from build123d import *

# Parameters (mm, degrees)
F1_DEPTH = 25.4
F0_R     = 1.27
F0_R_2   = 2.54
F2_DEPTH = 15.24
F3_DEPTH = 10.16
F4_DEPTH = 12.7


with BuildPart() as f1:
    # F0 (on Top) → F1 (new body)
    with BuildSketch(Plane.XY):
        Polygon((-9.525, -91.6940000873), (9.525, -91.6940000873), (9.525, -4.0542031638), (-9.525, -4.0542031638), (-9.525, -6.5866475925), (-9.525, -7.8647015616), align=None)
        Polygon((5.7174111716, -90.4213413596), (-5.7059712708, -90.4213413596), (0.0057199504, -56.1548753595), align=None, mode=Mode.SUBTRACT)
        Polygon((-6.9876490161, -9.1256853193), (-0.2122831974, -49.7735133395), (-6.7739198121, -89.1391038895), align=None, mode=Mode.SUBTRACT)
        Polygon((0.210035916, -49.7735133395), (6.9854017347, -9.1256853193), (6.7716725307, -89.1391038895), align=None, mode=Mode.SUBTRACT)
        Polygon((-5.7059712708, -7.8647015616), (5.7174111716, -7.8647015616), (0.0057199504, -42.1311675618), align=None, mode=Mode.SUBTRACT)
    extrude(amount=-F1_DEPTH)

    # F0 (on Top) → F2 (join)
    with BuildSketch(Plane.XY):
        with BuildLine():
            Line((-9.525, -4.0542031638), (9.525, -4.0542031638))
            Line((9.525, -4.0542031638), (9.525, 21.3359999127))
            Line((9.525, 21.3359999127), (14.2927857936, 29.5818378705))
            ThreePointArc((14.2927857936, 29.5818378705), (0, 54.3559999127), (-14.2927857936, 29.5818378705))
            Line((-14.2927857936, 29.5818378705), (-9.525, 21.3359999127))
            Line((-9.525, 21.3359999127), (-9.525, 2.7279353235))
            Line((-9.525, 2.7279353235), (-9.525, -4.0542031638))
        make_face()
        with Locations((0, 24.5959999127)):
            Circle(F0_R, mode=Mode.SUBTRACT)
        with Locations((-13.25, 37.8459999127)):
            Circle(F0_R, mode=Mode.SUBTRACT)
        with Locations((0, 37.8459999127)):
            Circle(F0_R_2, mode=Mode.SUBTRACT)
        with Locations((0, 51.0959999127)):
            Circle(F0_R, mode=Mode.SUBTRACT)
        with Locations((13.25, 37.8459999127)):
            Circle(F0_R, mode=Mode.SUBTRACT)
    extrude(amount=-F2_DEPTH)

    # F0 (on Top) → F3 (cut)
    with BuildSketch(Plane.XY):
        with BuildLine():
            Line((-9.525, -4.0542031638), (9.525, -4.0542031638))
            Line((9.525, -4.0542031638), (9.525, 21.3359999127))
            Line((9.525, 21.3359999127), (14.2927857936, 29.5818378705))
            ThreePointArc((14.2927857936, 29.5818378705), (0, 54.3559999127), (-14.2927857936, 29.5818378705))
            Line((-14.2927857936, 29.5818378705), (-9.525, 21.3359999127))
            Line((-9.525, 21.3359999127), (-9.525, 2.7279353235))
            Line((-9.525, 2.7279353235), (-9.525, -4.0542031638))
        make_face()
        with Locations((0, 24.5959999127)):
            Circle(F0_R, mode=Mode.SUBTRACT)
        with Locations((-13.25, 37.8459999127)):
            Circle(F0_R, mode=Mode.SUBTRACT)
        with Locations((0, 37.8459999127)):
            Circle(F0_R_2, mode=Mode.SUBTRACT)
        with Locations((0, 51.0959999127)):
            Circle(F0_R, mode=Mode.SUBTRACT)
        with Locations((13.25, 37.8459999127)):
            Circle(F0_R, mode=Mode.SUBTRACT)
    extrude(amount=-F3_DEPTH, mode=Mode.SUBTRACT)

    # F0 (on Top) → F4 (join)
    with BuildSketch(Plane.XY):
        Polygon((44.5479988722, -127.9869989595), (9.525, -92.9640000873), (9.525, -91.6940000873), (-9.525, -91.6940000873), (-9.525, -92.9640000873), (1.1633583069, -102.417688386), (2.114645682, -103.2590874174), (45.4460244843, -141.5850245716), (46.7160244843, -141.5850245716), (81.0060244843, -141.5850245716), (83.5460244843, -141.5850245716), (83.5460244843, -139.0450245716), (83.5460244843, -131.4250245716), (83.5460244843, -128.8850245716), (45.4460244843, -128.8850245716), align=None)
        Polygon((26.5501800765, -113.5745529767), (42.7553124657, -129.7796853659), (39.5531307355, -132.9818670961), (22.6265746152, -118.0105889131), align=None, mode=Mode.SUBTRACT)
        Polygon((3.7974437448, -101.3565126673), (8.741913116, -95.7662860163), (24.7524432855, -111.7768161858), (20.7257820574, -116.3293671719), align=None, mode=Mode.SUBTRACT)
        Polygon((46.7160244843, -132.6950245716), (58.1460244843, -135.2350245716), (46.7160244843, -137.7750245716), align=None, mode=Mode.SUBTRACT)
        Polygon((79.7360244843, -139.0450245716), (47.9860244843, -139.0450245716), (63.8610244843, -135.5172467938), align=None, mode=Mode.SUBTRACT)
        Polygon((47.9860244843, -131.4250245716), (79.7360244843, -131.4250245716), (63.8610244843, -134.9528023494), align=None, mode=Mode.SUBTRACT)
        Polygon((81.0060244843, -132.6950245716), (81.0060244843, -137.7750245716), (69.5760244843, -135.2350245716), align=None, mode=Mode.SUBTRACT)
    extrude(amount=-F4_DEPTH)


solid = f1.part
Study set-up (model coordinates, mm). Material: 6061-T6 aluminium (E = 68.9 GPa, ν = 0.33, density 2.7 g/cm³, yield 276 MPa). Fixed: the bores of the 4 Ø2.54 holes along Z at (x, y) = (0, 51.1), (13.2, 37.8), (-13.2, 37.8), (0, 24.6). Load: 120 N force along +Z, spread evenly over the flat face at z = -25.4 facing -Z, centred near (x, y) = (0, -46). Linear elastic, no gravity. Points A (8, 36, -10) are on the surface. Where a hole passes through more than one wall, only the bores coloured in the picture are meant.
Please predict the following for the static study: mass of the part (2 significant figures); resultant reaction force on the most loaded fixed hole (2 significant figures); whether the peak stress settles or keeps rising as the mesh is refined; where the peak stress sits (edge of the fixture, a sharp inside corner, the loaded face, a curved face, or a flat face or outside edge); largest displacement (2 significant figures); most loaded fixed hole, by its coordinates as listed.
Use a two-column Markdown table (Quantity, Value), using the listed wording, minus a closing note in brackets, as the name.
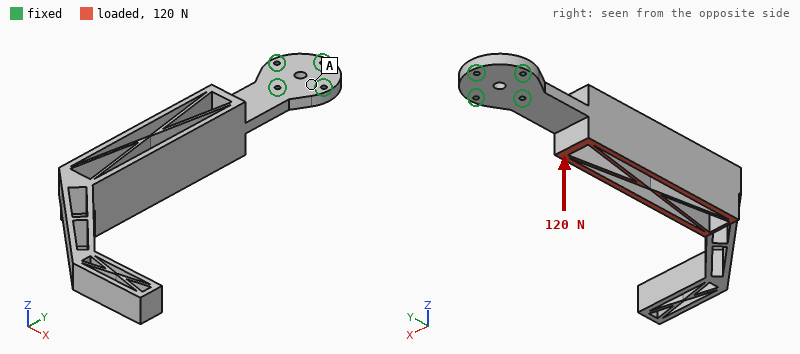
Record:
| Quantity | Value |
|---|---|
| mass of the part | 95 g |
| resultant reaction force on the most loaded fixed hole | 430 N |
| whether the peak stress settles or keeps rising as the mesh is refined | keeps rising |
| where the peak stress sits | edge of the fixture |
| largest displacement | 2.2 mm |
| most loaded fixed hole, by its coordinates as listed | (0, 24.6) |
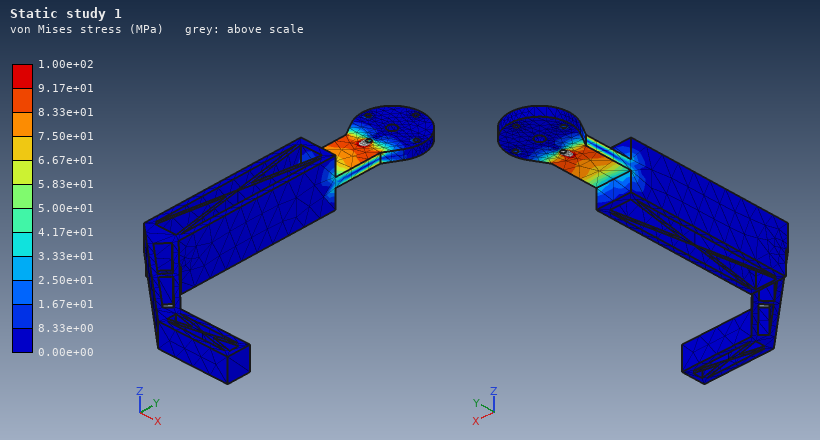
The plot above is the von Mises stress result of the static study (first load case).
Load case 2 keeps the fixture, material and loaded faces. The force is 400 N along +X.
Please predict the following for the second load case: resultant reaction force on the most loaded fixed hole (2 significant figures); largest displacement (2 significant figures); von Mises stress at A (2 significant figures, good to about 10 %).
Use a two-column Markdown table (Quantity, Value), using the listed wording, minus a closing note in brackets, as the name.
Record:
| Quantity | Value |
|---|---|
| resultant reaction force on the most loaded fixed hole | 860 N |
| largest displacement | 1.5 mm |
| von Mises stress at A | 23 MPa |
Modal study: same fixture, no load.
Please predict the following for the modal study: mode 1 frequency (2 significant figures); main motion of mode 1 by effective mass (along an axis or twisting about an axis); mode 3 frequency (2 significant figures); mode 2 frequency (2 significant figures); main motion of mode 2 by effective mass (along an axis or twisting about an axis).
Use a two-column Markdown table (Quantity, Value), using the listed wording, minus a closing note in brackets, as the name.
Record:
| Quantity | Value |
|---|---|
| mode 1 frequency | 130 Hz |
| main motion of mode 1 by effective mass | along Z |
| mode 3 frequency | 450 Hz |
| mode 2 frequency | 340 Hz |
| main motion of mode 2 by effective mass | along X |
